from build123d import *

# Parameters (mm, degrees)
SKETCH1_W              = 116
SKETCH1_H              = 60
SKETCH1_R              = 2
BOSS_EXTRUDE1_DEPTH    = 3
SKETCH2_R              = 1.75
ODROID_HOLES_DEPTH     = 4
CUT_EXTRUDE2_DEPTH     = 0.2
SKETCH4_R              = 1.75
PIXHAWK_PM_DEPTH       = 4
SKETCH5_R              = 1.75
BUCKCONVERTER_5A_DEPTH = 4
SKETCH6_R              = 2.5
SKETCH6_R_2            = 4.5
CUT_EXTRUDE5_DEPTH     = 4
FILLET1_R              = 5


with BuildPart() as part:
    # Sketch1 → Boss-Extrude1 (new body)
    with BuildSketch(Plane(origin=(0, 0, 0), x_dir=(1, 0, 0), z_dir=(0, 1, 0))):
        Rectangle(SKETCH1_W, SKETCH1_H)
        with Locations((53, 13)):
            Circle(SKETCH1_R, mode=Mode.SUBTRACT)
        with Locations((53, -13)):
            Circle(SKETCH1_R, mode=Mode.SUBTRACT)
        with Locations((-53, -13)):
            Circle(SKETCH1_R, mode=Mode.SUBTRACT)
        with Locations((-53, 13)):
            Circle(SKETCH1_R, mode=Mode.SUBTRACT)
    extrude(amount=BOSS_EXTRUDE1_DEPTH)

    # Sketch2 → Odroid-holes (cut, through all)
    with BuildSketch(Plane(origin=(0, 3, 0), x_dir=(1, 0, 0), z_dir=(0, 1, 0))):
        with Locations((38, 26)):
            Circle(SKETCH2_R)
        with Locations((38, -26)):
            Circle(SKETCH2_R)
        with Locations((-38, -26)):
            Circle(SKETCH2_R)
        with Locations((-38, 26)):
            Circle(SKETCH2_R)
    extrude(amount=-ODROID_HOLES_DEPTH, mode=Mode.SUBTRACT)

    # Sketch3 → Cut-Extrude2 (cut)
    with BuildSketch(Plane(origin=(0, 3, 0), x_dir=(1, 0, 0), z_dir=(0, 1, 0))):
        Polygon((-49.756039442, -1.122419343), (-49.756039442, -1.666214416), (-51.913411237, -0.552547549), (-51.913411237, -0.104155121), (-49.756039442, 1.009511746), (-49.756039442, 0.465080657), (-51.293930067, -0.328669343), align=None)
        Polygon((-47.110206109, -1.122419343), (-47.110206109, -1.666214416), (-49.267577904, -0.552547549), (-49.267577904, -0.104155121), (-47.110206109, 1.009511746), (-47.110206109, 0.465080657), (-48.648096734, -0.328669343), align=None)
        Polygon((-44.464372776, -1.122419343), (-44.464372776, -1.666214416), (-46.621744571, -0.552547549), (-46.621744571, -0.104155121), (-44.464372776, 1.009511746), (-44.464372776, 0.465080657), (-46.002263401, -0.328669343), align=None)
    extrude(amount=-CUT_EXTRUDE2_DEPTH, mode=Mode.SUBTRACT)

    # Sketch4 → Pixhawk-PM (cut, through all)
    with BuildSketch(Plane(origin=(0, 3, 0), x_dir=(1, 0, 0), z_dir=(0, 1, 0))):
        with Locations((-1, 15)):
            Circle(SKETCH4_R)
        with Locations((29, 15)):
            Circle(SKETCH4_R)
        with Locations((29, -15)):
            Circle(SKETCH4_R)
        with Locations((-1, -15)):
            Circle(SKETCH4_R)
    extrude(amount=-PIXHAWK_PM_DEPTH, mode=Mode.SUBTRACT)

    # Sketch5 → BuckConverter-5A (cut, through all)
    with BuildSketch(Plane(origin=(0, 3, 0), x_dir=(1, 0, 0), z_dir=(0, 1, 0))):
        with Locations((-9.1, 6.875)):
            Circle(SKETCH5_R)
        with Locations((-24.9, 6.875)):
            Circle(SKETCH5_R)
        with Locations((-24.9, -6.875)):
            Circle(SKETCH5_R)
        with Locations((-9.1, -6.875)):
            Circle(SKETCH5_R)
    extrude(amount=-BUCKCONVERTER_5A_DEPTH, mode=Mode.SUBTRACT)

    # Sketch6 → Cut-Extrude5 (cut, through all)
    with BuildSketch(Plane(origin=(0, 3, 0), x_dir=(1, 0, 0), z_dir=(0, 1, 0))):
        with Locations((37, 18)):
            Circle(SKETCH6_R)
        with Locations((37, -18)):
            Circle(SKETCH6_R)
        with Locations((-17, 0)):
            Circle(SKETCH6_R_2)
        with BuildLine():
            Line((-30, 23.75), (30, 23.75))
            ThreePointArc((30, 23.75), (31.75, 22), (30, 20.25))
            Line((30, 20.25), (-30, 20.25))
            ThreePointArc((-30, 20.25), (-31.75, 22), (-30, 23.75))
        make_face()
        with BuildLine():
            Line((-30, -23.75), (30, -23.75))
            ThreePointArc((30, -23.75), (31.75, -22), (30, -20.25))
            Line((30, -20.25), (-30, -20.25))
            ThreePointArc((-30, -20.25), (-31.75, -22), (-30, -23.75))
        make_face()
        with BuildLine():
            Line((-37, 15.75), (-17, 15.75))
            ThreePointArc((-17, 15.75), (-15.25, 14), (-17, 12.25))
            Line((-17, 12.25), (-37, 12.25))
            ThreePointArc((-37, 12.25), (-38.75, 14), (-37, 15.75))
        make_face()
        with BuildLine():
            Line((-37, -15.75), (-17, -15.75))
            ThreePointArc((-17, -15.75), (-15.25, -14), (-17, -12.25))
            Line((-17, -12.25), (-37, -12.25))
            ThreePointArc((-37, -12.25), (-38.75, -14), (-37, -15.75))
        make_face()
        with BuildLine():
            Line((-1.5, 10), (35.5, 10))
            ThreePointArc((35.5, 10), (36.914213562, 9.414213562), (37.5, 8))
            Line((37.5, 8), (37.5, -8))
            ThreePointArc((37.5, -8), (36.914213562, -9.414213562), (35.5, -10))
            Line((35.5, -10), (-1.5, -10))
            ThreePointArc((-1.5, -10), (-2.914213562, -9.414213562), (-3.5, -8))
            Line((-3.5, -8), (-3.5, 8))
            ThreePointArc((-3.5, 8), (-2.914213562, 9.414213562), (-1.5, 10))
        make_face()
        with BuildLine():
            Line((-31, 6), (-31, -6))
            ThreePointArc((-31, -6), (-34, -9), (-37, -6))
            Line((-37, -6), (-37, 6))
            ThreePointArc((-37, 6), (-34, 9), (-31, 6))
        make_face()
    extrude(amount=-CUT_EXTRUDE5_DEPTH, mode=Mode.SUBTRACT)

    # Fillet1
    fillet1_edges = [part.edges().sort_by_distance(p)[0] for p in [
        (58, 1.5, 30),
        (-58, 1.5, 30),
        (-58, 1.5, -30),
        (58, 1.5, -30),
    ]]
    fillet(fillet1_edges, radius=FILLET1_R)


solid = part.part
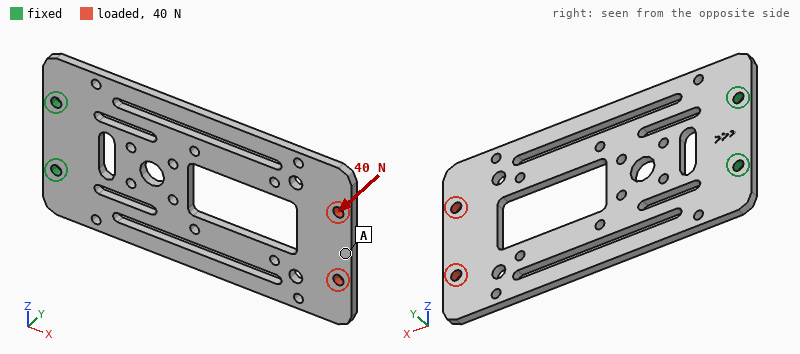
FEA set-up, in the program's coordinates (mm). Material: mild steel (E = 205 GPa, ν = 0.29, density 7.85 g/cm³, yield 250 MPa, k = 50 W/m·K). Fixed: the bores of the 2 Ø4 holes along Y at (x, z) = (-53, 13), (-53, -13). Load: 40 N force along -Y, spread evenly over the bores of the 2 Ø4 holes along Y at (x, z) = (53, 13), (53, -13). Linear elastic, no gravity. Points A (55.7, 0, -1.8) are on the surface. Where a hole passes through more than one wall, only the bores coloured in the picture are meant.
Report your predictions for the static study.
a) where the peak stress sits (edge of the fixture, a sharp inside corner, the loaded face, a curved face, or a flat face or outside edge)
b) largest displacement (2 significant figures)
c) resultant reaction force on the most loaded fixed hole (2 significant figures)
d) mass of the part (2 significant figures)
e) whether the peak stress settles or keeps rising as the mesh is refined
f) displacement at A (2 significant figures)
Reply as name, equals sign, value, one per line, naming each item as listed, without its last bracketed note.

where the peak stress sits = edge of the fixture
largest displacement = 0.98 mm
resultant reaction force on the most loaded fixed hole = 20 N
mass of the part = 120 g
whether the peak stress settles or keeps rising as the mesh is refined = keeps rising
displacement at A = 0.95 mm
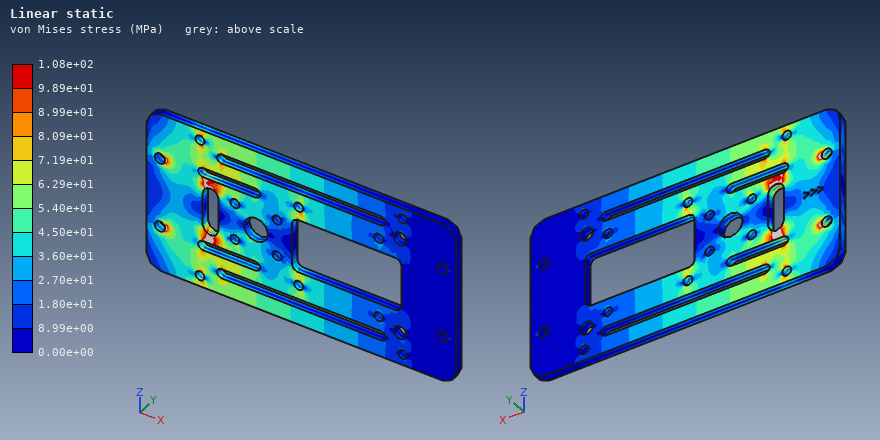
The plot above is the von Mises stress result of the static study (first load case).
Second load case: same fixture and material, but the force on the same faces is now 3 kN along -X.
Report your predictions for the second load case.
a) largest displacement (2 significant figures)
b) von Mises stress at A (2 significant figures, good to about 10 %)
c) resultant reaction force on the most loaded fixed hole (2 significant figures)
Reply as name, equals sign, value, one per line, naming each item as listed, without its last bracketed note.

largest displacement = 22 µm
von Mises stress at A = 18 MPa
resultant reaction force on the most loaded fixed hole = 1.5 kN
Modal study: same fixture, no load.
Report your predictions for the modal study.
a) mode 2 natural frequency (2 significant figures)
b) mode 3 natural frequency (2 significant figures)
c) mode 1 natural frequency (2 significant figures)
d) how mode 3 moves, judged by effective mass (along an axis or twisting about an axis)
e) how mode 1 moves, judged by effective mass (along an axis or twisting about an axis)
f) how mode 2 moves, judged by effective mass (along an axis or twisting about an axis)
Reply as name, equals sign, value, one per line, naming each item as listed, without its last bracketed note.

mode 2 natural frequency = 650 Hz
mode 3 natural frequency = 1200 Hz
mode 1 natural frequency = 180 Hz
how mode 3 moves, judged by effective mass = along Y
how mode 1 moves, judged by effective mass = along Y
how mode 2 moves, judged by effective mass = twisting about X
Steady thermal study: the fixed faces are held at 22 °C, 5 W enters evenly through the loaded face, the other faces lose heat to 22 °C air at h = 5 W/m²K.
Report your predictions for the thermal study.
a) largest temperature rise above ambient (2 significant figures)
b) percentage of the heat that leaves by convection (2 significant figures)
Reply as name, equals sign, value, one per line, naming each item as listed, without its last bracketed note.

largest temperature rise above ambient = 74 K
percentage of the heat that leaves by convection = 43 %
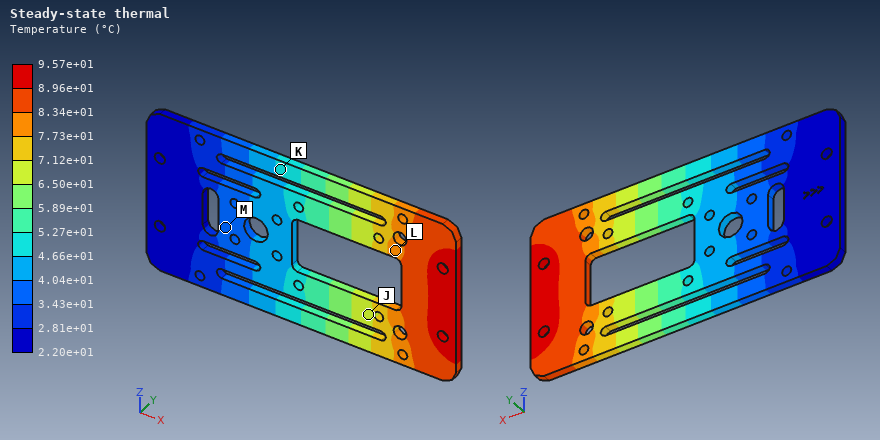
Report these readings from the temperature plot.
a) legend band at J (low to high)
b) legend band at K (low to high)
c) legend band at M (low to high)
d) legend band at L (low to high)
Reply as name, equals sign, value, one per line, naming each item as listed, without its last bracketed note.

legend band at J = 6.50e+01 to 7.12e+01 °C
legend band at K = 4.66e+01 to 5.27e+01 °C
legend band at M = 3.43e+01 to 4.04e+01 °C
legend band at L = 7.73e+01 to 8.34e+01 °C
